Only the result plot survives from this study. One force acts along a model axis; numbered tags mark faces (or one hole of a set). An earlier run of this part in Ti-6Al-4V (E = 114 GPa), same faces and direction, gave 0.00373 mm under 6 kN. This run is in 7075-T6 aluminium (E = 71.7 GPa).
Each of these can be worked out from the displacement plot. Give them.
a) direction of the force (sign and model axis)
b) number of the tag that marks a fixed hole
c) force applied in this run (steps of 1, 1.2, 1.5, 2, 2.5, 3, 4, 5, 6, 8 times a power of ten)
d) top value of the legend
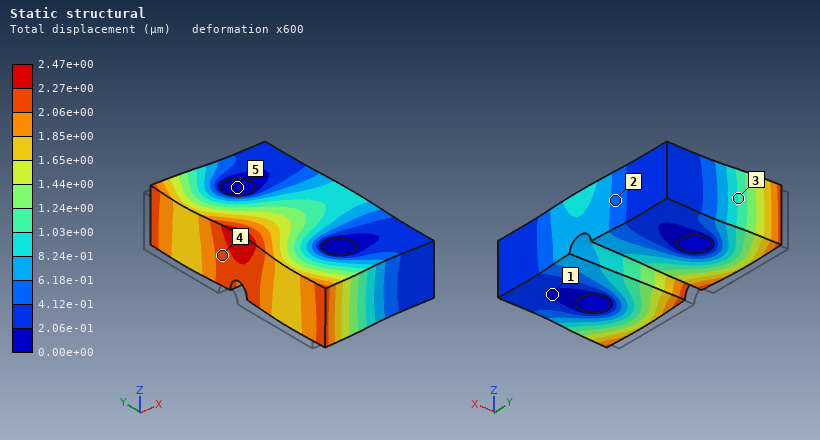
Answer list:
+X
5
2.5 kN
2.47e+00 µm
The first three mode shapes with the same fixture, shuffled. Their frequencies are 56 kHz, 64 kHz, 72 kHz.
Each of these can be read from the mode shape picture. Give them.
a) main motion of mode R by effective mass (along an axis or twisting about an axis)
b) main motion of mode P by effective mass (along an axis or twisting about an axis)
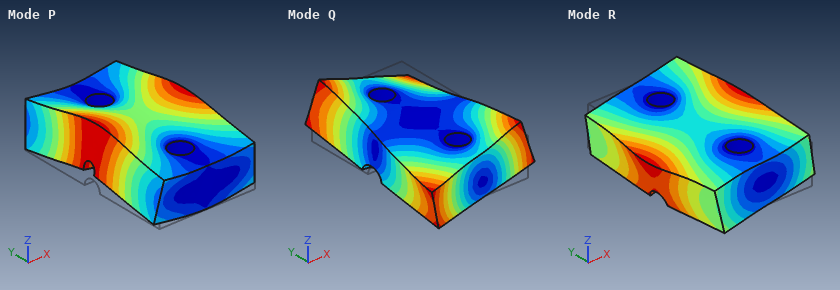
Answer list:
twisting about Y
along Z
